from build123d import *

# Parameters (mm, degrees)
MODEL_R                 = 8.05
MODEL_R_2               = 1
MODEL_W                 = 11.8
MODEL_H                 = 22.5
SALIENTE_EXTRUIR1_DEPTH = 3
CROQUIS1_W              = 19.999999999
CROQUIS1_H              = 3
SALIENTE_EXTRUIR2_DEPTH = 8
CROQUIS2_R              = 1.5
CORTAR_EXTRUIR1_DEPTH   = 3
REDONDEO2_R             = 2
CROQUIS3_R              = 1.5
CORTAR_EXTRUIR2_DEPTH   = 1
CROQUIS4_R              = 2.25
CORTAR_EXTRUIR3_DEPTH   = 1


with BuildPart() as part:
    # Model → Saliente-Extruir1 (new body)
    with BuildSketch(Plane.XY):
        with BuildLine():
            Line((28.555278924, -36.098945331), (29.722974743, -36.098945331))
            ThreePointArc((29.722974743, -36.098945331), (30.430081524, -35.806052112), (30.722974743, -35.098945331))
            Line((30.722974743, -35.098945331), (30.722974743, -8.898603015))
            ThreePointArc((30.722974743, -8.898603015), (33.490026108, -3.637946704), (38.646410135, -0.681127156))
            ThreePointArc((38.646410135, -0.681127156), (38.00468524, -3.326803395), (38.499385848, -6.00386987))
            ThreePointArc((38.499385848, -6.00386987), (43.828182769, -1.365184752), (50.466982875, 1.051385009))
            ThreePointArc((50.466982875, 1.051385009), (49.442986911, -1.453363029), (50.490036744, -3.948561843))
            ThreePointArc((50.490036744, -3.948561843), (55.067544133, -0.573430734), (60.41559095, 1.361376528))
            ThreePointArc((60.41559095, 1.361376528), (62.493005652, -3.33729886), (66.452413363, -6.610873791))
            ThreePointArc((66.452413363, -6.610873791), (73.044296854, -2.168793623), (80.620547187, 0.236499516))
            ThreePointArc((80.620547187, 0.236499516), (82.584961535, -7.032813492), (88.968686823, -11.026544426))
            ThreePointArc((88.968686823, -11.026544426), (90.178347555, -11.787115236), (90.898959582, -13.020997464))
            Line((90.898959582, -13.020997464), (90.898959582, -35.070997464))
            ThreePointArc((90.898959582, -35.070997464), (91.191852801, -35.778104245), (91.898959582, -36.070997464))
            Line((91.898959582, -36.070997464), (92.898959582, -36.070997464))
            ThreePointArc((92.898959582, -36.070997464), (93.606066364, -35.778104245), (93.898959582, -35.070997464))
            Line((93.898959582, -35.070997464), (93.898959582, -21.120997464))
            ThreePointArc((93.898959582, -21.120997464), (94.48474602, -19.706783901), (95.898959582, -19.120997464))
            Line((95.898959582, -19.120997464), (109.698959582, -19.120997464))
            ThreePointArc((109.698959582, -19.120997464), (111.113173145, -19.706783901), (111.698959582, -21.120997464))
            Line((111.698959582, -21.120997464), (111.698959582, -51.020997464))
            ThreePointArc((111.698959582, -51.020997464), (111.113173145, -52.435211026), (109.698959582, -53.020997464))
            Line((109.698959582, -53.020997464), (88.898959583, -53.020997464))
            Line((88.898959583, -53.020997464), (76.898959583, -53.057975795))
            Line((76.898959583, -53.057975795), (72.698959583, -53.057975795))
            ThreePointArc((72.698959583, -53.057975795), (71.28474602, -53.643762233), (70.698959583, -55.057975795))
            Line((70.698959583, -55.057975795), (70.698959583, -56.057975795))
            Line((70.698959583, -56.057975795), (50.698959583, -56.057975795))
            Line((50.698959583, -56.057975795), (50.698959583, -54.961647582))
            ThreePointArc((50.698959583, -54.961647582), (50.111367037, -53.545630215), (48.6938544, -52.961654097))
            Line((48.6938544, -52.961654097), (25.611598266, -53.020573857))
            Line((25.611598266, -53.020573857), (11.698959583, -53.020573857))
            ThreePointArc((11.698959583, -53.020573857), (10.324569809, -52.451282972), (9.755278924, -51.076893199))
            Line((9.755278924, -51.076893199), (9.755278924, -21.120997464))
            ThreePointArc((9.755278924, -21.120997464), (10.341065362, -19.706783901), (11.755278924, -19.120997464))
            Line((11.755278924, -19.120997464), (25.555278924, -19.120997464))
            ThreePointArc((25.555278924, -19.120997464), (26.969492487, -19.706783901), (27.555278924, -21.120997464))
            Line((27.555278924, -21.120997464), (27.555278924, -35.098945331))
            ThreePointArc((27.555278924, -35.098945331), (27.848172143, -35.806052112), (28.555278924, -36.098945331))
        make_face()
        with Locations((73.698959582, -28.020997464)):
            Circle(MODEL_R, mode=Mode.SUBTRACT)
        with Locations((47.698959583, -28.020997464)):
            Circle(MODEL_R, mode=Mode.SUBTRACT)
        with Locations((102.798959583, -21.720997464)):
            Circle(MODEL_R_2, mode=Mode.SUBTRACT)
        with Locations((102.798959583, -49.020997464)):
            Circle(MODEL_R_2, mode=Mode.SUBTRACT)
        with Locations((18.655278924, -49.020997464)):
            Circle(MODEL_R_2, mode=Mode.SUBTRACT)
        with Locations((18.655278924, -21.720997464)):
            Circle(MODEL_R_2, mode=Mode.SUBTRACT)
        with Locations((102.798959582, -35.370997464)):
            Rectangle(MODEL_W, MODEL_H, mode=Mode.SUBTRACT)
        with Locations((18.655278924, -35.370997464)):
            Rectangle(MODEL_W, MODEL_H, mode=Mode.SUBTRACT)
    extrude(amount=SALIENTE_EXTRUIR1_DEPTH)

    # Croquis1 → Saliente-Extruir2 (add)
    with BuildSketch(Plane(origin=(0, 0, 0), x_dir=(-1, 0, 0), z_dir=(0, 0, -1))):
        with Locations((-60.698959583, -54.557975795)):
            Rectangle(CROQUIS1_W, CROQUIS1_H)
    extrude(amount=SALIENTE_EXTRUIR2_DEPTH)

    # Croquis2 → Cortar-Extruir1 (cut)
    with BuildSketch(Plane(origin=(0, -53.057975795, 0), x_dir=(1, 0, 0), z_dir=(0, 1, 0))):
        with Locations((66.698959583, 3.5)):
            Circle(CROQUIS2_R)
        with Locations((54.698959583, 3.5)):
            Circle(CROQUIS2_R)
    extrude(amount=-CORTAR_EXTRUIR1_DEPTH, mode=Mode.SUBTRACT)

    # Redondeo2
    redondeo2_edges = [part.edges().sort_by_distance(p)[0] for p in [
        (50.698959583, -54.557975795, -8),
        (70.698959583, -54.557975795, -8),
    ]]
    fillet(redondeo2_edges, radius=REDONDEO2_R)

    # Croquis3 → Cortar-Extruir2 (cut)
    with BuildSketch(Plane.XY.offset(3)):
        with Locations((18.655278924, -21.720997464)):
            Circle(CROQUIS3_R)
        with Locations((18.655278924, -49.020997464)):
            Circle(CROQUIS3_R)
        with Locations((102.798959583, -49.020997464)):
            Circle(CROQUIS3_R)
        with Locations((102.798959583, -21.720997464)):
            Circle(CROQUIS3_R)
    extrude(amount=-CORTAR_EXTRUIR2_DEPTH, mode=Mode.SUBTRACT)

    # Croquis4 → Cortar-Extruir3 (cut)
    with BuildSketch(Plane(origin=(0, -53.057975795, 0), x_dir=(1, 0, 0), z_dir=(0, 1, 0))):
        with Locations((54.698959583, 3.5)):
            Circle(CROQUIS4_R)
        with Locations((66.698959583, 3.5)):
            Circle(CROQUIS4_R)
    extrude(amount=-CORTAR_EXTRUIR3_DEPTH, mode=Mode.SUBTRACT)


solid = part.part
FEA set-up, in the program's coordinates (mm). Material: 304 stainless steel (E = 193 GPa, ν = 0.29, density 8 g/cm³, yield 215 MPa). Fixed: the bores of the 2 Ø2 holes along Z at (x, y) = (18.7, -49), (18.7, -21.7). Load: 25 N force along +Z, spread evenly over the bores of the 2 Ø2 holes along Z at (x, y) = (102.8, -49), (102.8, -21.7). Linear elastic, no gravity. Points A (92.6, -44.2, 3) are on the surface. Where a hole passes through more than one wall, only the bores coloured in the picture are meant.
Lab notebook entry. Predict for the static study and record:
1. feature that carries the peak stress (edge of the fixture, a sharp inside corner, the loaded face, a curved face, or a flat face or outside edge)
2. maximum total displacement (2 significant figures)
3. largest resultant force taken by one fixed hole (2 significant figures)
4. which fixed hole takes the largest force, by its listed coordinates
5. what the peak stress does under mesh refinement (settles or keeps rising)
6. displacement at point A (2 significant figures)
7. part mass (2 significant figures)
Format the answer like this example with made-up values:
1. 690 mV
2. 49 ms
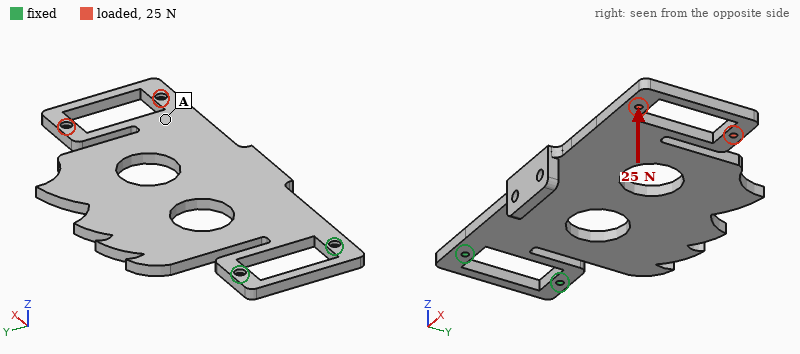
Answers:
1. edge of the fixture
2. 1.0 mm
3. 16 N
4. (18.7, -21.7)
5. keeps rising
6. 0.71 mm
7. 85 g
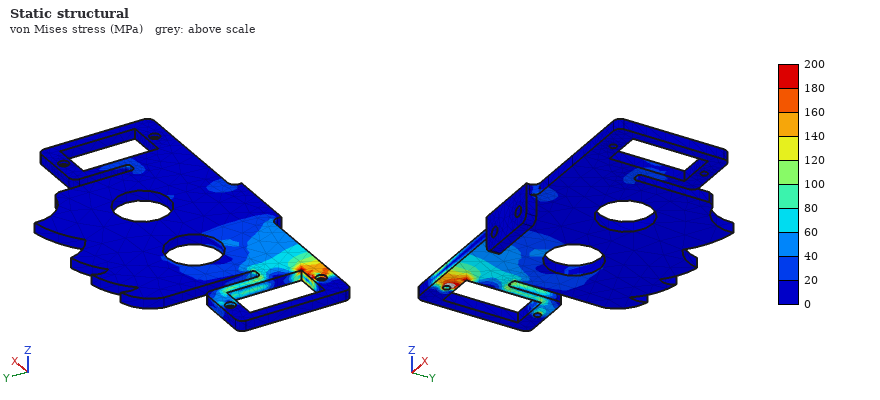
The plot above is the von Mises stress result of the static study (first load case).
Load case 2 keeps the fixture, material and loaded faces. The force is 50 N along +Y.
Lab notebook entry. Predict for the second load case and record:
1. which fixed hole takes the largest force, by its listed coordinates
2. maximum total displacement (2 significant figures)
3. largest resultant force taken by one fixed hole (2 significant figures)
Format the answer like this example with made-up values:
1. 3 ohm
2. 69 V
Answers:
1. (18.7, -21.7)
2. 0.13 mm
3. 190 N
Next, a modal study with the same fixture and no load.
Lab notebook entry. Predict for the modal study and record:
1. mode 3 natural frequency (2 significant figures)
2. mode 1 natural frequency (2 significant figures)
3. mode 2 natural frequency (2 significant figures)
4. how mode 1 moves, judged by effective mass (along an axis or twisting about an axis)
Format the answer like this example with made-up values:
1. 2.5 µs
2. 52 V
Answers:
1. 610 Hz
2. 180 Hz
3. 590 Hz
4. along Z
